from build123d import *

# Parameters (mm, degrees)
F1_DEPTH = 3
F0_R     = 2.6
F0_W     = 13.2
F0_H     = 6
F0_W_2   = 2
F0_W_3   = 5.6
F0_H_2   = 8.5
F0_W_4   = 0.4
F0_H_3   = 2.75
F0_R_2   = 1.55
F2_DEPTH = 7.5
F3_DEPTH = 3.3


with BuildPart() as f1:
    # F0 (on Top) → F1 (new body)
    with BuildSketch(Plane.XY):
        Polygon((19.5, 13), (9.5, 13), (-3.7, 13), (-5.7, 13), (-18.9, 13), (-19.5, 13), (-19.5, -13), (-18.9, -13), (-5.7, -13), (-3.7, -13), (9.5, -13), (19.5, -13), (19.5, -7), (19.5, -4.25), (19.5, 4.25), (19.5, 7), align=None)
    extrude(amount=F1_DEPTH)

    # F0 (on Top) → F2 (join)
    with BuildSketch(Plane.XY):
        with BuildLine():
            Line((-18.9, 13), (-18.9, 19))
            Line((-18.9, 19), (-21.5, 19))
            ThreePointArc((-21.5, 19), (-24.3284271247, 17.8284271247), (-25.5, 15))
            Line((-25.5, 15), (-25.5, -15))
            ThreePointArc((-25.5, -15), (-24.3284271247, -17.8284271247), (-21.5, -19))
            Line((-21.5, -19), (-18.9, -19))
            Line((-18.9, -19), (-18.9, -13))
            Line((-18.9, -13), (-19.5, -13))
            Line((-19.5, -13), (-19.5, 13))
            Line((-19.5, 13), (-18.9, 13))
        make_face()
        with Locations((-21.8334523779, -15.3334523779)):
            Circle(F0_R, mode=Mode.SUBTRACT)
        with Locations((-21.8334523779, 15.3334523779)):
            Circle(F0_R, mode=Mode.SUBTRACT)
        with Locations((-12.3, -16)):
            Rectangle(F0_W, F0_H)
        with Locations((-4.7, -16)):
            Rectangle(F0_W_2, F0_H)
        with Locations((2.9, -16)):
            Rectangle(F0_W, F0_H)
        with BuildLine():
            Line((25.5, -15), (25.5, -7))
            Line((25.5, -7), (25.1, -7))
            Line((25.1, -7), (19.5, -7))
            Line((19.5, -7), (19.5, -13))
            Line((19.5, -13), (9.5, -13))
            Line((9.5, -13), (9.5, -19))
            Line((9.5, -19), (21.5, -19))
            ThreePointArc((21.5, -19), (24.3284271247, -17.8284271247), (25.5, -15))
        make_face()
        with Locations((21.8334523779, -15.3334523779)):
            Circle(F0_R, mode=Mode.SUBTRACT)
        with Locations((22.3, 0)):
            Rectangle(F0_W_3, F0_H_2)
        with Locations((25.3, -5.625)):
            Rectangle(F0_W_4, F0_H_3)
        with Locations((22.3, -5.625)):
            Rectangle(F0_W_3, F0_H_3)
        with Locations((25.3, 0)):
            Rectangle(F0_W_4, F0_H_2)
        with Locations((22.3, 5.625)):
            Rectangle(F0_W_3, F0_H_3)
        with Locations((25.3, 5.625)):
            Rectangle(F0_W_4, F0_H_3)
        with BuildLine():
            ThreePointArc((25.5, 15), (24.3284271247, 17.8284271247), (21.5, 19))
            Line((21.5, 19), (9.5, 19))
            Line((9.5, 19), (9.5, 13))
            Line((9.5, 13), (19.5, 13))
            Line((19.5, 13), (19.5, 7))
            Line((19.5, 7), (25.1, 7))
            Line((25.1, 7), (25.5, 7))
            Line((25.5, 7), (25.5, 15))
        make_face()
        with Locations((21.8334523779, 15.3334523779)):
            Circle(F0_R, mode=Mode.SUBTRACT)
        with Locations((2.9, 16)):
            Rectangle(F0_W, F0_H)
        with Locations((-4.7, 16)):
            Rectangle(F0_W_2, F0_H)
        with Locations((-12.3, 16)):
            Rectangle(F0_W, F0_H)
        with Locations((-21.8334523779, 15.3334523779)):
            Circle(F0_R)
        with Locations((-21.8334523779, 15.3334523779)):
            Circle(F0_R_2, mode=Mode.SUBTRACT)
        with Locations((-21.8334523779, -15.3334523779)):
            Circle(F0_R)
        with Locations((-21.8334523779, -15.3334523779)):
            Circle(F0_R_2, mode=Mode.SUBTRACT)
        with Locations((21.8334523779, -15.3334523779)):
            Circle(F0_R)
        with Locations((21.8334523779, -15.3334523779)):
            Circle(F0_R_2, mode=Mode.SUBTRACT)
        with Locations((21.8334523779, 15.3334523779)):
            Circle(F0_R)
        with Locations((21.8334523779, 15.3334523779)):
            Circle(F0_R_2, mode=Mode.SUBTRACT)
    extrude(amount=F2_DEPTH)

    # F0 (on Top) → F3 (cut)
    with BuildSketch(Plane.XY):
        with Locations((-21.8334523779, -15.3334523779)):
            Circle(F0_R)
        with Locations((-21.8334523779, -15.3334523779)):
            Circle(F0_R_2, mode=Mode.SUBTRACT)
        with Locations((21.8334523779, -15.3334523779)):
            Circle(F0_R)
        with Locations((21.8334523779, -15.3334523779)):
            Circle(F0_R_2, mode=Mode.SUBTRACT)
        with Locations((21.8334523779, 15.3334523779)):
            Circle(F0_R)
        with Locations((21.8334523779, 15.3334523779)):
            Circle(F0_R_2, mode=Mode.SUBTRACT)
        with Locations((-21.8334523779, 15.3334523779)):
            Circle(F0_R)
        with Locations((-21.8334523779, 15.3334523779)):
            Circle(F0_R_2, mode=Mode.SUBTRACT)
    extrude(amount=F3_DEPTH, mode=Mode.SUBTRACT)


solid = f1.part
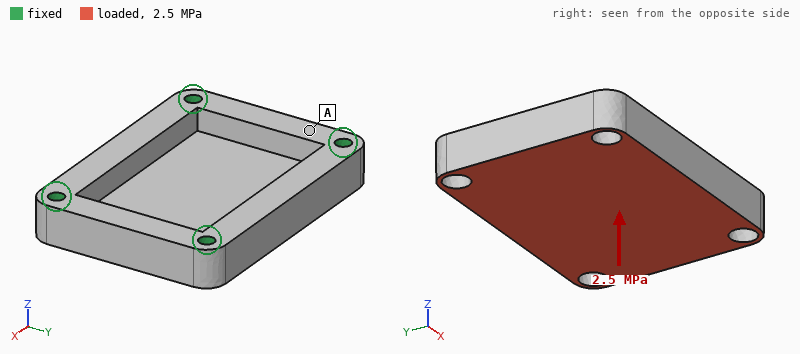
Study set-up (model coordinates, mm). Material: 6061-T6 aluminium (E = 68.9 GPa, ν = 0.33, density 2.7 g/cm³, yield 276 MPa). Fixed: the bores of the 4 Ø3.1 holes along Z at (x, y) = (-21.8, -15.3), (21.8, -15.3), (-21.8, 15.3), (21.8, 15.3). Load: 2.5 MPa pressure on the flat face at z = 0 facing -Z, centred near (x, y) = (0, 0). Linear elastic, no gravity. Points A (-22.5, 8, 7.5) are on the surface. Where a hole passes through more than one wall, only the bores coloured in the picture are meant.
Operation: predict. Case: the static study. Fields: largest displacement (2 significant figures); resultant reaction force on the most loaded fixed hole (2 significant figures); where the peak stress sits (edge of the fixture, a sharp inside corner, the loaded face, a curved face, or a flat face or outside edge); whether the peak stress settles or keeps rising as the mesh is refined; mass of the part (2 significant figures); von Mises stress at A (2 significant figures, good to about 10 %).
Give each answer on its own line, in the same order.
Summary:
73 µm
1.6 kN
edge of the fixture
keeps rising
26 g
29 MPa
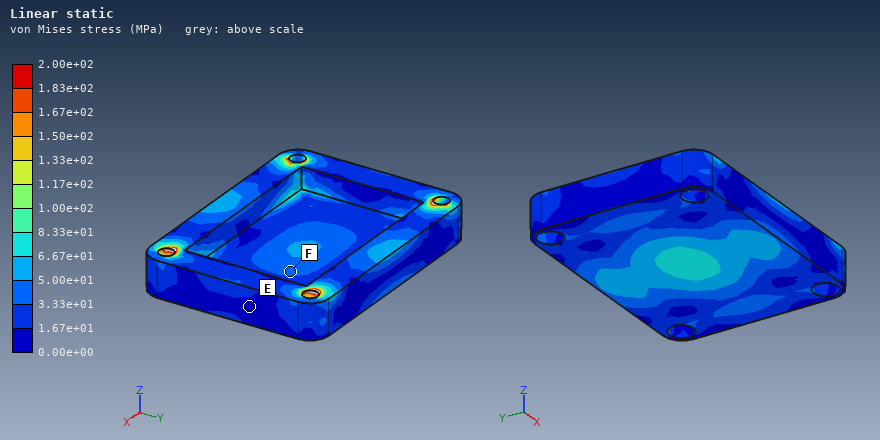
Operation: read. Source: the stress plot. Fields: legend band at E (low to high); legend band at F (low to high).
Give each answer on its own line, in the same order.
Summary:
0.00e+00 to 1.67e+01 MPa
3.33e+01 to 5.00e+01 MPa
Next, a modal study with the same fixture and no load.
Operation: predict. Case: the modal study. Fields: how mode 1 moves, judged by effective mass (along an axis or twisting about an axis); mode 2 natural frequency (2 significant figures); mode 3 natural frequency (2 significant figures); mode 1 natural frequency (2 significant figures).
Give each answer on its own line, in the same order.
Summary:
along Z
15 kHz
19 kHz
12 kHz
